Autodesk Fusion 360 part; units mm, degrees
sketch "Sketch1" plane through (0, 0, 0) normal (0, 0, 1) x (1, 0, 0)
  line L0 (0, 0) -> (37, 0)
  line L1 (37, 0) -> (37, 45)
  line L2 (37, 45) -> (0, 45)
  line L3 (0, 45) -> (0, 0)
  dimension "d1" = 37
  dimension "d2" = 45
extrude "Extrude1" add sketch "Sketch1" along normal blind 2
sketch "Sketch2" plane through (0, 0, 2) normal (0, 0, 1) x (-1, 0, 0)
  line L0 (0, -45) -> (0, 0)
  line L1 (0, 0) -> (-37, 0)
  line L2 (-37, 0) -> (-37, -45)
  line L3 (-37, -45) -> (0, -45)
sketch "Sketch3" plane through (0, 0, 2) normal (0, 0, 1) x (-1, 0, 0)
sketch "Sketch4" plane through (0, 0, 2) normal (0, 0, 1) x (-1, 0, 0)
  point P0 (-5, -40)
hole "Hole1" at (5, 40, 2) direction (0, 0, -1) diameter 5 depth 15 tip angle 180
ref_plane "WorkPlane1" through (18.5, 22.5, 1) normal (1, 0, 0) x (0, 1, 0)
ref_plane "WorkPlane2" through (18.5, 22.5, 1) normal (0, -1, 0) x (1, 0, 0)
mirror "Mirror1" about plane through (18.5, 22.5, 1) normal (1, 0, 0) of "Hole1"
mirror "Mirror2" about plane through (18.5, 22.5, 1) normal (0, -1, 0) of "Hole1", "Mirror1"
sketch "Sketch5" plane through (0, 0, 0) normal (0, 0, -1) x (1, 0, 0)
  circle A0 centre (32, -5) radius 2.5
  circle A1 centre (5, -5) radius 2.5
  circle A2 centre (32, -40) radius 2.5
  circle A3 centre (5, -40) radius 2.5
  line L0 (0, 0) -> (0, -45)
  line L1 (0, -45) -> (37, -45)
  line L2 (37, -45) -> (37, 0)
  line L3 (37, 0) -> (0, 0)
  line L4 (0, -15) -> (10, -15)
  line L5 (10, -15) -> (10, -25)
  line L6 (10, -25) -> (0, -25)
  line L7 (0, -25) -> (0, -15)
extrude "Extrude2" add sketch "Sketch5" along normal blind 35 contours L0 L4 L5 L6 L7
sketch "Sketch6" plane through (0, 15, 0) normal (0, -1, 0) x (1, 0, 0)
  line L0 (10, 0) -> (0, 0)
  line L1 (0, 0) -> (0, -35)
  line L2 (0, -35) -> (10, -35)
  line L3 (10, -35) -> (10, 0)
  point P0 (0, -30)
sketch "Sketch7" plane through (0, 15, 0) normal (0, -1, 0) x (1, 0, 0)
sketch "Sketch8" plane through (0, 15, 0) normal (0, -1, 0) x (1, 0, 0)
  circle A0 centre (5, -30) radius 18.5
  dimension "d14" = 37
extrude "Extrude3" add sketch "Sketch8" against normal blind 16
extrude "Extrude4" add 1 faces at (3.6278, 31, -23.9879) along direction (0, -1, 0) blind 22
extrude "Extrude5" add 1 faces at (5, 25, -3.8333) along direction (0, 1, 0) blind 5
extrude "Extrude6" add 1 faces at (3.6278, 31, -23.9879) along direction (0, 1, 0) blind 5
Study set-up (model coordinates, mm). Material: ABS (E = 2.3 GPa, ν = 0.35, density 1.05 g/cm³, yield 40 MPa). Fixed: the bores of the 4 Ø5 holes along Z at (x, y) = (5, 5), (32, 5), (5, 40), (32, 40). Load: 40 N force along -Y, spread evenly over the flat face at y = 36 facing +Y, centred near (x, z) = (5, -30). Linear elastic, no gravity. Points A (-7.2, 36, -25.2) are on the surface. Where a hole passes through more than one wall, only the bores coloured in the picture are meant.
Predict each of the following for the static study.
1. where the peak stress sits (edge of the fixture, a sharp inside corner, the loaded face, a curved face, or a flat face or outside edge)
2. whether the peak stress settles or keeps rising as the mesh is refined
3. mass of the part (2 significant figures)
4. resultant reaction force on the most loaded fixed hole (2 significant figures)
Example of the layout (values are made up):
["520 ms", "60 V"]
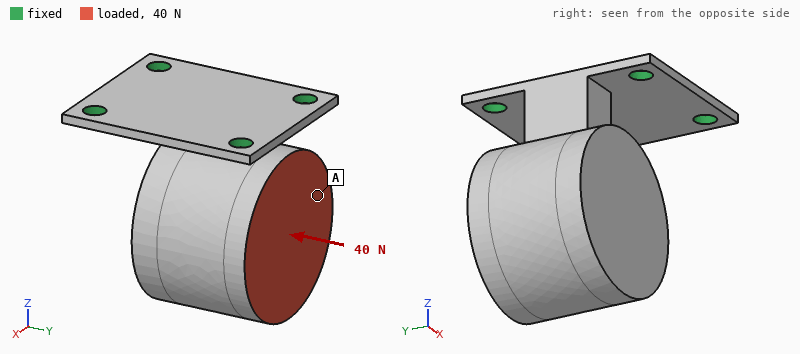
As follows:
["edge of the fixture", "keeps rising", "36 g", "52 N"]
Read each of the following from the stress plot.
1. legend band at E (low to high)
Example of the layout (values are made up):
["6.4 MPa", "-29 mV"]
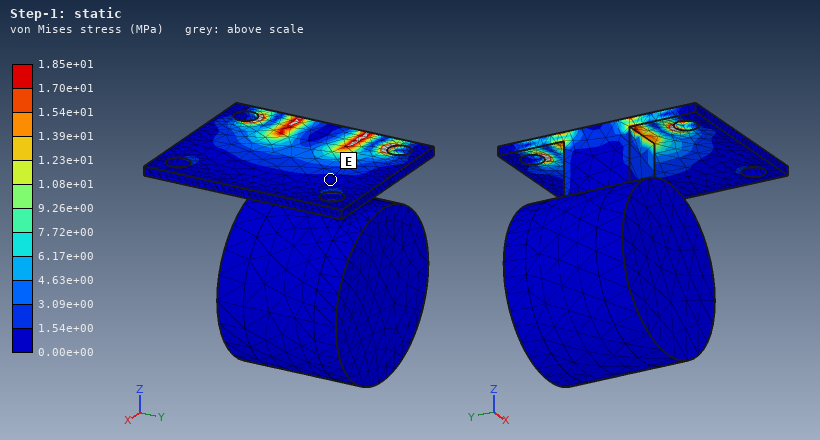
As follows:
["0.00e+00 to 1.54e+00 MPa"]
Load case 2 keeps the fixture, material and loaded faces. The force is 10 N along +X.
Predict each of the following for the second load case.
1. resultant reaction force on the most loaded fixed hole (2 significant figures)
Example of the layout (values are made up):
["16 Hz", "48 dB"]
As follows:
["8.0 N"]
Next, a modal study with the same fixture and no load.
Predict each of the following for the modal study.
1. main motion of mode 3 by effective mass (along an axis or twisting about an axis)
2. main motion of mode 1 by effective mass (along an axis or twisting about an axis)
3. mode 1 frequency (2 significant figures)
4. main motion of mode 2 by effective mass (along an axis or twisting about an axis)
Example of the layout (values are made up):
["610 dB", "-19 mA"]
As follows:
["along Z", "along X", "110 Hz", "along Y"]
